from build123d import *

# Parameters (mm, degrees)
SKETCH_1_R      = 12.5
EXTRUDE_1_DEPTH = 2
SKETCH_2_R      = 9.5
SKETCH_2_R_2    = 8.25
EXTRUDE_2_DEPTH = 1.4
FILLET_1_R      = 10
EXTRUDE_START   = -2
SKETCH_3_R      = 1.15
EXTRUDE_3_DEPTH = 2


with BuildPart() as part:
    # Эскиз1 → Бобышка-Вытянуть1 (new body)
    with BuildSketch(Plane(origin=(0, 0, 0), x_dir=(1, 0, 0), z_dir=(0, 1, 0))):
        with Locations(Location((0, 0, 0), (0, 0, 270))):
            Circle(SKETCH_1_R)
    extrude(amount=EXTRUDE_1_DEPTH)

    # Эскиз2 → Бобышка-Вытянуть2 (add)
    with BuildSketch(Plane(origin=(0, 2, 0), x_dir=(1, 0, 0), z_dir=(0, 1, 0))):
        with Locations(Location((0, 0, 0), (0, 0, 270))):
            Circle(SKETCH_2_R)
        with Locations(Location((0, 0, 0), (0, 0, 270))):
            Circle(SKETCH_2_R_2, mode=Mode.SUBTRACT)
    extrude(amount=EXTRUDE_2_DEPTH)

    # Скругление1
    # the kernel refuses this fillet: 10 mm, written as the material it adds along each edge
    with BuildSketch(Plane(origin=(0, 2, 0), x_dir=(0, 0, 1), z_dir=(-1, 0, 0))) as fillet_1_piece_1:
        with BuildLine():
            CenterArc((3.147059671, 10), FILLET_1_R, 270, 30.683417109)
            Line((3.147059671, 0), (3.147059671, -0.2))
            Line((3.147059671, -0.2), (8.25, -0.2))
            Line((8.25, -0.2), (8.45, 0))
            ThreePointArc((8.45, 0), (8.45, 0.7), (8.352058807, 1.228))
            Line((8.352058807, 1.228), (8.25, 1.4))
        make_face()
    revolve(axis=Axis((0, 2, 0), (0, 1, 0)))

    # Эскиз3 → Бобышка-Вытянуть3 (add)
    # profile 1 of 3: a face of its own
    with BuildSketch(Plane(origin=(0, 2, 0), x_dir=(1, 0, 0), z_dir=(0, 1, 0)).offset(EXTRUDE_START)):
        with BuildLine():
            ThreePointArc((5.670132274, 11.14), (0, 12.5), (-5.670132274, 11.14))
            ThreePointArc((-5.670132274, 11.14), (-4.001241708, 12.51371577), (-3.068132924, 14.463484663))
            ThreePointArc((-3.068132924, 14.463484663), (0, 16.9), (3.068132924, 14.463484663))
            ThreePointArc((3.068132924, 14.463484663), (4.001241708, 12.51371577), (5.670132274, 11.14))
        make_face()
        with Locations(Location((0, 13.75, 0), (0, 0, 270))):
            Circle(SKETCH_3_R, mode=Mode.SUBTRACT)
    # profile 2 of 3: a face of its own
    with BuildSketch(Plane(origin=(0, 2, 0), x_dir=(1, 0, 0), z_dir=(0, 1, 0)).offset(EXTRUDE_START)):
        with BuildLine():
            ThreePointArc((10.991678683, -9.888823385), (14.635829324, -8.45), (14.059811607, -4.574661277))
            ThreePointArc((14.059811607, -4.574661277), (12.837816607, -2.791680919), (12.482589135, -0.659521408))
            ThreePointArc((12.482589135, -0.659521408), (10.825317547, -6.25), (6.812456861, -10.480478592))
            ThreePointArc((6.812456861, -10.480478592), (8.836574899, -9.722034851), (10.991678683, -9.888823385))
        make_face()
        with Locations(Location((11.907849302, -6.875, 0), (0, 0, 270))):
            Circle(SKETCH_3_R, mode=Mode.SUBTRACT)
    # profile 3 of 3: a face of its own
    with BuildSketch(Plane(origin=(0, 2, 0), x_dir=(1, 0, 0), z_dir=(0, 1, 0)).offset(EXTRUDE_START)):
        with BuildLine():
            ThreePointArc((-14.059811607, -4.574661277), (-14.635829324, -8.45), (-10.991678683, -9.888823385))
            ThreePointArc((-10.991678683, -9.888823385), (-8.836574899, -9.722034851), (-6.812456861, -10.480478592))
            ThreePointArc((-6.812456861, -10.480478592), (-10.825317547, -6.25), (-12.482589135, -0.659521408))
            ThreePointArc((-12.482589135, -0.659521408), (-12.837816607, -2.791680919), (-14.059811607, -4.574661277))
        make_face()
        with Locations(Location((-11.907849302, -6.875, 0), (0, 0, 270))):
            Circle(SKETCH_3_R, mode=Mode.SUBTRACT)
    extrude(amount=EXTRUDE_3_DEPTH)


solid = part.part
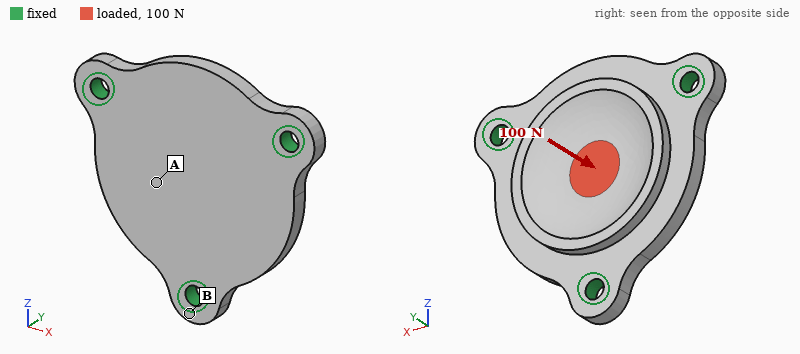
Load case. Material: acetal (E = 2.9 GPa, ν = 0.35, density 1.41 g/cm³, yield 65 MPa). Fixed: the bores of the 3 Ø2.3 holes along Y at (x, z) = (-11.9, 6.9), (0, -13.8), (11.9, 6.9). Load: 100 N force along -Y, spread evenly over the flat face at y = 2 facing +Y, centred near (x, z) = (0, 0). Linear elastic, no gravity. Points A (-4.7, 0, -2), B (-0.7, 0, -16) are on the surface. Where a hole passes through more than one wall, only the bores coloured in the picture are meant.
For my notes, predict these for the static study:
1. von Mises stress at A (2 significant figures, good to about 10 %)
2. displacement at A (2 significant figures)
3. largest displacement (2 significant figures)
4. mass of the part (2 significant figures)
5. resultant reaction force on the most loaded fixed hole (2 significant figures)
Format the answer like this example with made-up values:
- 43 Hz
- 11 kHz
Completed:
- 11 MPa
- 0.13 mm
- 0.18 mm
- 1.9 g
- 37 N
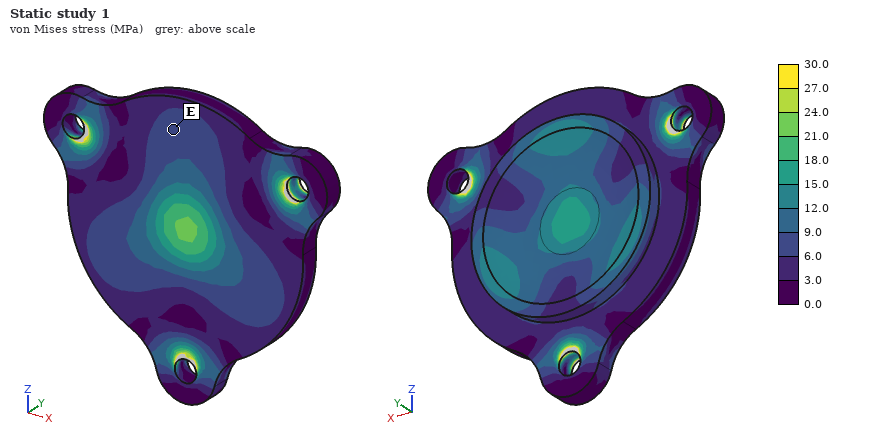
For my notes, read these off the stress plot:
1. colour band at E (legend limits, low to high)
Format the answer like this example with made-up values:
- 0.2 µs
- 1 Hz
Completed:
- 6.0 to 9.0 MPa
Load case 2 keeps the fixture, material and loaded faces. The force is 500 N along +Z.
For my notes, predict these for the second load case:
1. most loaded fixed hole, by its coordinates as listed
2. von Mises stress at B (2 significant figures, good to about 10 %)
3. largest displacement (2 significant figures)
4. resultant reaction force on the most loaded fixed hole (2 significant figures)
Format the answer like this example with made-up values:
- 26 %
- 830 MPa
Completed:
- (0, -13.8)
- 6.7 MPa
- 0.10 mm
- 230 N
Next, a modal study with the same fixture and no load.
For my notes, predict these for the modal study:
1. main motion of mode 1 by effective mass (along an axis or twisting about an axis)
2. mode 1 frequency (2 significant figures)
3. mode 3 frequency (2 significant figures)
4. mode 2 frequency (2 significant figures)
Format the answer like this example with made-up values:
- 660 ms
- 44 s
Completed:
- along Y
- 4900 Hz
- 5500 Hz
- 5500 Hz
